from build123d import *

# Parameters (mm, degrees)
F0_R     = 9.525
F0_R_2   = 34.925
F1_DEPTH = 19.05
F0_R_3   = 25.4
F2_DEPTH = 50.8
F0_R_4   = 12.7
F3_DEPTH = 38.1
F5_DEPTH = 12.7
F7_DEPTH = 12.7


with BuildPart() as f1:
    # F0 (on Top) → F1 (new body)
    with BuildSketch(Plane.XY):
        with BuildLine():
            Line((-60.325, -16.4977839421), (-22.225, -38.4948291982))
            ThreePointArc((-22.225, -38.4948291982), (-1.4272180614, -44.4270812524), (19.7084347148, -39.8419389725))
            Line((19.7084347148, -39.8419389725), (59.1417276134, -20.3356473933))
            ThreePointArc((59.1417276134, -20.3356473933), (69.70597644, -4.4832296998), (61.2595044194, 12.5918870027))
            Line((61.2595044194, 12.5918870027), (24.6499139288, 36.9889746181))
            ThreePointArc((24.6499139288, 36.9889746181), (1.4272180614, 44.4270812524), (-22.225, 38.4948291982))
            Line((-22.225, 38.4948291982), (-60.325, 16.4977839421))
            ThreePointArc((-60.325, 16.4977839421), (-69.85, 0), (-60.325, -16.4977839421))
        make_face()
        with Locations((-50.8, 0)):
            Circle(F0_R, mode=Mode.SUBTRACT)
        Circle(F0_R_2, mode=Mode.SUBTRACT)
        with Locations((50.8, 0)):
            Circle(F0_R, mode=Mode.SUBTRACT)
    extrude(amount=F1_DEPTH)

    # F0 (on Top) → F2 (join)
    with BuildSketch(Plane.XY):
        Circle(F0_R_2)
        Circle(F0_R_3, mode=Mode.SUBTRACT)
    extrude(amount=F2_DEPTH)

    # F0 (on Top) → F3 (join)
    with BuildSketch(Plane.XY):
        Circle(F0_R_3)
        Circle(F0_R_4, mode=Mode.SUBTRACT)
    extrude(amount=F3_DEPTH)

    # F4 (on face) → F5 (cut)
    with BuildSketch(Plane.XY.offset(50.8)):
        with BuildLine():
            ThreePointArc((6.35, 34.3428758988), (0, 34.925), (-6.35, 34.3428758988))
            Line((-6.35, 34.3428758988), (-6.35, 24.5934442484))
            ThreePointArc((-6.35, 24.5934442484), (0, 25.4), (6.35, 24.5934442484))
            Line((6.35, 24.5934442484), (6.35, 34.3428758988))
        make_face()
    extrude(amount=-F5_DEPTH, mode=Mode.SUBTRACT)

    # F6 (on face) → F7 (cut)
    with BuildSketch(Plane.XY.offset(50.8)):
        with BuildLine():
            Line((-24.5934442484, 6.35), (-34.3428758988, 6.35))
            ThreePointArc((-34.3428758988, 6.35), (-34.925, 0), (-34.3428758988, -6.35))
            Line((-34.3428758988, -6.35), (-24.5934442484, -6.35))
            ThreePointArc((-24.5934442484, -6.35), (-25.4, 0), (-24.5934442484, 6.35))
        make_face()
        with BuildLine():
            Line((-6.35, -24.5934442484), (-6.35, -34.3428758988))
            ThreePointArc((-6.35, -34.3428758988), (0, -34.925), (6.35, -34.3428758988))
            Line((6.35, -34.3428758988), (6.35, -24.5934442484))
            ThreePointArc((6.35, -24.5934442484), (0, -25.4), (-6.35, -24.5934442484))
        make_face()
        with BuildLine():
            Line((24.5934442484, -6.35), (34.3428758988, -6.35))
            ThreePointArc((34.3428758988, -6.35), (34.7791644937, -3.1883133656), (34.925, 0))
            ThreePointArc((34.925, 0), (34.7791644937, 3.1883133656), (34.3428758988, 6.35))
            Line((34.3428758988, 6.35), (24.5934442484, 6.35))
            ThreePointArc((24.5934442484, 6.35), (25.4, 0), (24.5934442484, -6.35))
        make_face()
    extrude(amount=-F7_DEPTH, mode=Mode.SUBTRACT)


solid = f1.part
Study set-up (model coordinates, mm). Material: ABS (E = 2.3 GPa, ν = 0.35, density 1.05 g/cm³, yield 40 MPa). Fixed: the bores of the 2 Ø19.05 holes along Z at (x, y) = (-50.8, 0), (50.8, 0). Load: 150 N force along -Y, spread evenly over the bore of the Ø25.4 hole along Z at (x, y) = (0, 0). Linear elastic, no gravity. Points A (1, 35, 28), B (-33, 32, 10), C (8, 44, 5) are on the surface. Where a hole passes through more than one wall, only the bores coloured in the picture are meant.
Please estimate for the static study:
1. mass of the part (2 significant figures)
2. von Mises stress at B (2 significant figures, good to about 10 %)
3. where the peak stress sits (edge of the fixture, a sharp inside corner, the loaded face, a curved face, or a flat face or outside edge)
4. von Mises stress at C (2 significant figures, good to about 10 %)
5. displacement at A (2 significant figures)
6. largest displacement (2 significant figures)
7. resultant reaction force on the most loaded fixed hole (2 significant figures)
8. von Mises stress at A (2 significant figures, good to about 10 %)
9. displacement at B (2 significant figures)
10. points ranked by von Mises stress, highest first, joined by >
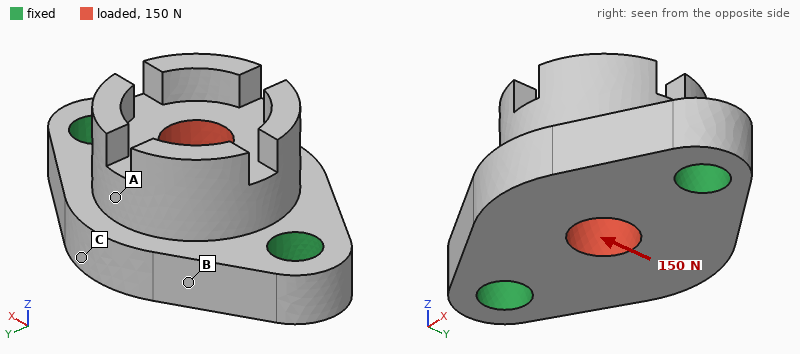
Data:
230 g
0.13 MPa
edge of the fixture
0.070 MPa
7.2 µm
9.7 µm
75 N
0.039 MPa
3.8 µm
B > C > A
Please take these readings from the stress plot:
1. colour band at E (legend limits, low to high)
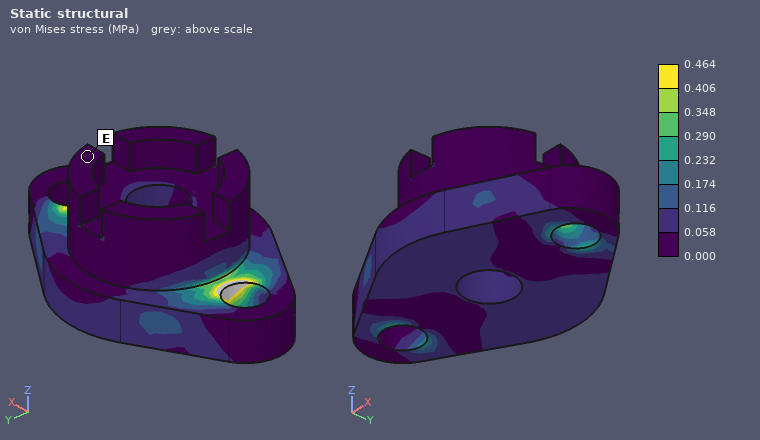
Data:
0.000 to 0.058 MPa
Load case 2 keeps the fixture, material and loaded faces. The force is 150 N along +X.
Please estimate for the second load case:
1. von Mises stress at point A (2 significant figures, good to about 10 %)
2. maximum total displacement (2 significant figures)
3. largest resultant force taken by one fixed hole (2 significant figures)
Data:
0.018 MPa
2.0 µm
77 N
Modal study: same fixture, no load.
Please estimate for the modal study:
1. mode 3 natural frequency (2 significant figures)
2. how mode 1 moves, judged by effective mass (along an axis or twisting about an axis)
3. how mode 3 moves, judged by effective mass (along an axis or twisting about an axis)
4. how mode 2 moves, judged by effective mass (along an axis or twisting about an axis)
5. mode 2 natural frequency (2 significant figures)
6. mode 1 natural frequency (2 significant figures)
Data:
3200 Hz
along Y
along Y
along Z
2100 Hz
1300 Hz
